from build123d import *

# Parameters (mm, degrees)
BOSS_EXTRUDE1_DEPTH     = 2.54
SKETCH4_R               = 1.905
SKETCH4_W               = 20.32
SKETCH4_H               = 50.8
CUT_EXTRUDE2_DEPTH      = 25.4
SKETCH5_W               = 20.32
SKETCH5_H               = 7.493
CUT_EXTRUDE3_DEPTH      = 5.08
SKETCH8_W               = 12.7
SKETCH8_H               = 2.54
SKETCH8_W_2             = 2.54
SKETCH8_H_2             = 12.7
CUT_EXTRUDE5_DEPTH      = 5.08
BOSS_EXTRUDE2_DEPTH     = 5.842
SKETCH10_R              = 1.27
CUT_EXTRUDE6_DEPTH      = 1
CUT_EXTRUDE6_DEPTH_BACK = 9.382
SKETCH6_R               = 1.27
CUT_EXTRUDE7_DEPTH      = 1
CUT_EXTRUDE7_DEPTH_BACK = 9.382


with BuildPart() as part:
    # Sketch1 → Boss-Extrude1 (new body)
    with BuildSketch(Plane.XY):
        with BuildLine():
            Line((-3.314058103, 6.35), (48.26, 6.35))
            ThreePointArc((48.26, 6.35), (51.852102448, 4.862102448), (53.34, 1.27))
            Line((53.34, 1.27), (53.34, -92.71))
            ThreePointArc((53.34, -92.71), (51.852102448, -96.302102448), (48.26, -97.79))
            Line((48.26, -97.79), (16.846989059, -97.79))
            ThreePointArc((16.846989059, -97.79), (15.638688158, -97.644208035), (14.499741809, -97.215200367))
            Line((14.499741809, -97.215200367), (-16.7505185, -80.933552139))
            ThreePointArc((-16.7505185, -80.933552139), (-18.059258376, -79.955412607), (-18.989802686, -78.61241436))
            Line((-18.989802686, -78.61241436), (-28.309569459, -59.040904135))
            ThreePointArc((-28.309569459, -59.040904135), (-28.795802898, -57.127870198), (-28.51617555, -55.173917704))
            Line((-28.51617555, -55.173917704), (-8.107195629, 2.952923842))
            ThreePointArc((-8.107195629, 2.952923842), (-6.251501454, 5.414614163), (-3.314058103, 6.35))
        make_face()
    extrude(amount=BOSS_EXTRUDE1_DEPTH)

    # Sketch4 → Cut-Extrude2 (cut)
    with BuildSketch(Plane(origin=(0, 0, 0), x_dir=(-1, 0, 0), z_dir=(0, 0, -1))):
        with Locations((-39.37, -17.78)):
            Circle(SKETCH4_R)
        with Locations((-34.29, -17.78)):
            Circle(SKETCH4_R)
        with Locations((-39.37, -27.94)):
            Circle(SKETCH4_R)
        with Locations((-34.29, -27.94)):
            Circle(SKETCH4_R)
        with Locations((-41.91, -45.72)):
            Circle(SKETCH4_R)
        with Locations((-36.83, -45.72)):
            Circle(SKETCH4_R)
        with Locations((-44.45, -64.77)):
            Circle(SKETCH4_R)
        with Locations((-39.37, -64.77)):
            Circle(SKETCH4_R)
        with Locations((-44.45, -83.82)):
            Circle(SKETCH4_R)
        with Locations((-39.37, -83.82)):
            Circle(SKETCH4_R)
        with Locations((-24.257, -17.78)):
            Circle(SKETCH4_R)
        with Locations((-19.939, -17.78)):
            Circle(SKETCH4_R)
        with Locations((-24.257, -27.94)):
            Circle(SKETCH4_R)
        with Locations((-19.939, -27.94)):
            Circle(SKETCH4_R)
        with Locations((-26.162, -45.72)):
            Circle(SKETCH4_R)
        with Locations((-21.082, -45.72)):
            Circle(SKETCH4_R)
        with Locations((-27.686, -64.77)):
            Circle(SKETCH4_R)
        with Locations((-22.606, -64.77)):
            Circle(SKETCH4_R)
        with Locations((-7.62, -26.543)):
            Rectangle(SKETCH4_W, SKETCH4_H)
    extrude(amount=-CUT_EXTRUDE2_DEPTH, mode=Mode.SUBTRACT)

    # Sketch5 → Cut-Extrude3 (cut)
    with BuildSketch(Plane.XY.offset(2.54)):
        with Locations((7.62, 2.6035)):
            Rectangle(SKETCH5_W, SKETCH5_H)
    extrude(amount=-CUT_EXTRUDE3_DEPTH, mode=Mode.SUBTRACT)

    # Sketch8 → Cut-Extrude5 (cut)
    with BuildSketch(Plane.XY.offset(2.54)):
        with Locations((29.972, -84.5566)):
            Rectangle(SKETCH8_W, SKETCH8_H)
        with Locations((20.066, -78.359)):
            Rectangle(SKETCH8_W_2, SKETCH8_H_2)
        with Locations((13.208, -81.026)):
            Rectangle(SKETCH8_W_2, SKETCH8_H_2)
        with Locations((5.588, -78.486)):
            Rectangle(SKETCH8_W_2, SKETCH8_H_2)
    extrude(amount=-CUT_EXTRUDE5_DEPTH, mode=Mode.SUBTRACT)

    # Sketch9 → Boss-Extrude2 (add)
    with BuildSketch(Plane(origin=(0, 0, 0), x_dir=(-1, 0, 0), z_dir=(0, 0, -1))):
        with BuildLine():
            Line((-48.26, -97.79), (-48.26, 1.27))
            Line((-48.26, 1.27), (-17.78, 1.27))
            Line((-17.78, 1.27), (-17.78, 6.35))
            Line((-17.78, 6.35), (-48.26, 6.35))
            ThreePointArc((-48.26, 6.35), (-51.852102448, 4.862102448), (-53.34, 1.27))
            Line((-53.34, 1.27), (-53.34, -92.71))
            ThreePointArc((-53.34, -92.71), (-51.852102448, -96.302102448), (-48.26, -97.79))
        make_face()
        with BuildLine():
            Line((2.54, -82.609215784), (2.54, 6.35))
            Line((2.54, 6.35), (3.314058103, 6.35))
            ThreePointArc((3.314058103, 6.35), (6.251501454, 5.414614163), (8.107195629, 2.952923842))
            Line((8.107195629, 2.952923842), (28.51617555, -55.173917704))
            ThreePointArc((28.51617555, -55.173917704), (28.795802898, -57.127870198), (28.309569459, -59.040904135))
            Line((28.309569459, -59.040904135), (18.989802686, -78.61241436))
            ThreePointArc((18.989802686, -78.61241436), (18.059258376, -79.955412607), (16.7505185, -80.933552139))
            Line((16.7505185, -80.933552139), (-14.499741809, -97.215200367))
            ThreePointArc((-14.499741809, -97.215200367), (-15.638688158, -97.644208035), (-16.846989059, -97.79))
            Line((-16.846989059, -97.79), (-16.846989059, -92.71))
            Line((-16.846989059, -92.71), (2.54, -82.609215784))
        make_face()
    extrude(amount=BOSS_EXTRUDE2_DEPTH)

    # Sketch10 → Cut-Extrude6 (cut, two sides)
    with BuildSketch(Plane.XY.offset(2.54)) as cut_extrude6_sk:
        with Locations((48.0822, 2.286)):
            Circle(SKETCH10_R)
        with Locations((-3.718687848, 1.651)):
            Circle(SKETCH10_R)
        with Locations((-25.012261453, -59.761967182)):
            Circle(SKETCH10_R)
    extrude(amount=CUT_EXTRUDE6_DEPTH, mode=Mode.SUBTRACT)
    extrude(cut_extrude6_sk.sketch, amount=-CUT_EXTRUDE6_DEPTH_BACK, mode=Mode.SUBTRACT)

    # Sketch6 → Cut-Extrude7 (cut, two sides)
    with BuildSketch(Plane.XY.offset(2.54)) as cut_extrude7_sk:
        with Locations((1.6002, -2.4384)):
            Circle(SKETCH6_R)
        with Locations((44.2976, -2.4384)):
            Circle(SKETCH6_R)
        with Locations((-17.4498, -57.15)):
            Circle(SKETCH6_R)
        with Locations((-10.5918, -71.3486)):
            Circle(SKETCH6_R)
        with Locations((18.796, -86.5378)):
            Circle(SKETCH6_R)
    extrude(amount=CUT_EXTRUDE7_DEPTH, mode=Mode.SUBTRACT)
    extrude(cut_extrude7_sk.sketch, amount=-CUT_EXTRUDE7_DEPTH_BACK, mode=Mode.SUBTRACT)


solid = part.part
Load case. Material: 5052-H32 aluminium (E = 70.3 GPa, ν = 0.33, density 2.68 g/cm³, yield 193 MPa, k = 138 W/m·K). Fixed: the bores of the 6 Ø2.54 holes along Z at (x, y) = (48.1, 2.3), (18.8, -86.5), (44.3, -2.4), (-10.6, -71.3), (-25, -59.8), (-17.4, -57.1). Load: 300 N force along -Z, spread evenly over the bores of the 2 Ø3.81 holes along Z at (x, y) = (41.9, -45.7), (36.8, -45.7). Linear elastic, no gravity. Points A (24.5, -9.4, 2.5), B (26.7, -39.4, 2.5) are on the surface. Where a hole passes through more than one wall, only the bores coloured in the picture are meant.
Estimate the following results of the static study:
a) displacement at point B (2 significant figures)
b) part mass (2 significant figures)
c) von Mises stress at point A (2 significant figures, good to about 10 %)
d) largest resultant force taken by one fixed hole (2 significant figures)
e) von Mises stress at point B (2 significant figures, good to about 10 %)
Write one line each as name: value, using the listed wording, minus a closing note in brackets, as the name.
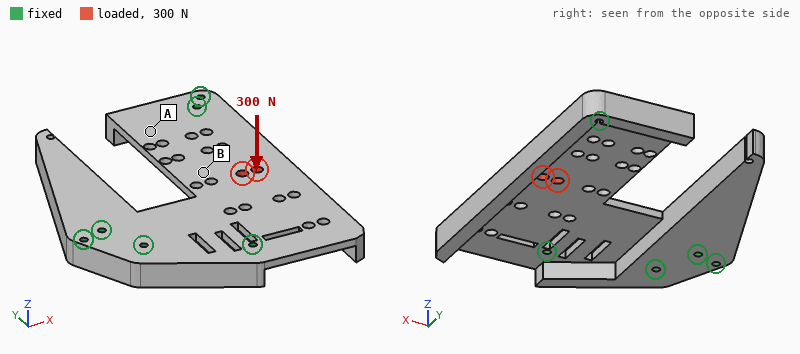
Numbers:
displacement at point B: 0.10 mm
part mass: 75 g
von Mises stress at point A: 8.7 MPa
largest resultant force taken by one fixed hole: 490 N
von Mises stress at point B: 23 MPa
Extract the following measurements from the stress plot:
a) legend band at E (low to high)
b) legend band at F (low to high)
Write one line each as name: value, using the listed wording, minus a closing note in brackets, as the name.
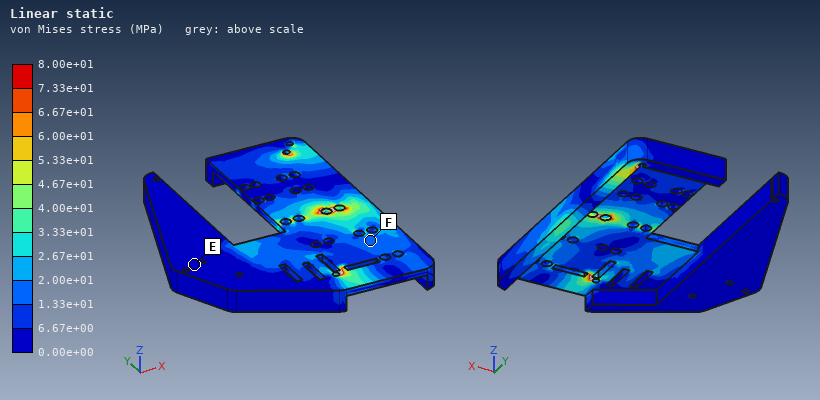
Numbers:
legend band at E: 0.00e+00 to 6.67e+00 MPa
legend band at F: 1.33e+01 to 2.00e+01 MPa
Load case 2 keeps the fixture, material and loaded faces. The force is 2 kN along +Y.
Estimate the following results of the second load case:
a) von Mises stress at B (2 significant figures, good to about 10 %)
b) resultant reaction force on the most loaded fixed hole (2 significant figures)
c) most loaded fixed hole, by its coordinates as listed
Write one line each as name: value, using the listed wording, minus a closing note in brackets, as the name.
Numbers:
von Mises stress at B: 8.5 MPa
resultant reaction force on the most loaded fixed hole: 800 N
most loaded fixed hole, by its coordinates as listed: (44.3, -2.4)
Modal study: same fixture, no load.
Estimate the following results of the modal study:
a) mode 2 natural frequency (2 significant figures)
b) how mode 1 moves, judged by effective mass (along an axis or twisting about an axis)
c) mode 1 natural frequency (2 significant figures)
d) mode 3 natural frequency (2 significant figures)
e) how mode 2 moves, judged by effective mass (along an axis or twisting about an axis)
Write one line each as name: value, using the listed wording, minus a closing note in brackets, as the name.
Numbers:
mode 2 natural frequency: 2500 Hz
how mode 1 moves, judged by effective mass: along Z
mode 1 natural frequency: 1500 Hz
mode 3 natural frequency: 3000 Hz
how mode 2 moves, judged by effective mass: along Z
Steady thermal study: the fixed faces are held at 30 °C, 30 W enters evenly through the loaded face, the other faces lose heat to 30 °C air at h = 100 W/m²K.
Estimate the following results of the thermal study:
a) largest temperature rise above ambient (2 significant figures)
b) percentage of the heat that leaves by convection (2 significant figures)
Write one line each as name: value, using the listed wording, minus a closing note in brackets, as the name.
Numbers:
largest temperature rise above ambient: 54 K
percentage of the heat that leaves by convection: 51 %
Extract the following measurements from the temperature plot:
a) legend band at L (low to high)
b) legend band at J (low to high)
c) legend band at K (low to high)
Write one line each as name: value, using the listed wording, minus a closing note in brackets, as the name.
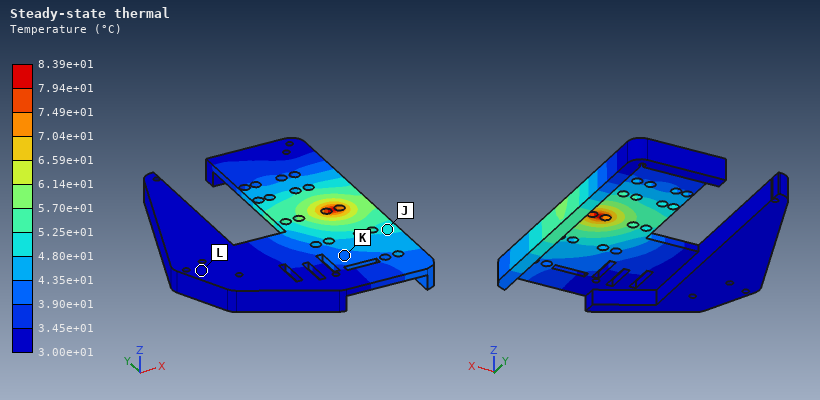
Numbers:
legend band at L: 3.00e+01 to 3.45e+01 °C
legend band at J: 4.80e+01 to 5.25e+01 °C
legend band at K: 3.90e+01 to 4.35e+01 °C
